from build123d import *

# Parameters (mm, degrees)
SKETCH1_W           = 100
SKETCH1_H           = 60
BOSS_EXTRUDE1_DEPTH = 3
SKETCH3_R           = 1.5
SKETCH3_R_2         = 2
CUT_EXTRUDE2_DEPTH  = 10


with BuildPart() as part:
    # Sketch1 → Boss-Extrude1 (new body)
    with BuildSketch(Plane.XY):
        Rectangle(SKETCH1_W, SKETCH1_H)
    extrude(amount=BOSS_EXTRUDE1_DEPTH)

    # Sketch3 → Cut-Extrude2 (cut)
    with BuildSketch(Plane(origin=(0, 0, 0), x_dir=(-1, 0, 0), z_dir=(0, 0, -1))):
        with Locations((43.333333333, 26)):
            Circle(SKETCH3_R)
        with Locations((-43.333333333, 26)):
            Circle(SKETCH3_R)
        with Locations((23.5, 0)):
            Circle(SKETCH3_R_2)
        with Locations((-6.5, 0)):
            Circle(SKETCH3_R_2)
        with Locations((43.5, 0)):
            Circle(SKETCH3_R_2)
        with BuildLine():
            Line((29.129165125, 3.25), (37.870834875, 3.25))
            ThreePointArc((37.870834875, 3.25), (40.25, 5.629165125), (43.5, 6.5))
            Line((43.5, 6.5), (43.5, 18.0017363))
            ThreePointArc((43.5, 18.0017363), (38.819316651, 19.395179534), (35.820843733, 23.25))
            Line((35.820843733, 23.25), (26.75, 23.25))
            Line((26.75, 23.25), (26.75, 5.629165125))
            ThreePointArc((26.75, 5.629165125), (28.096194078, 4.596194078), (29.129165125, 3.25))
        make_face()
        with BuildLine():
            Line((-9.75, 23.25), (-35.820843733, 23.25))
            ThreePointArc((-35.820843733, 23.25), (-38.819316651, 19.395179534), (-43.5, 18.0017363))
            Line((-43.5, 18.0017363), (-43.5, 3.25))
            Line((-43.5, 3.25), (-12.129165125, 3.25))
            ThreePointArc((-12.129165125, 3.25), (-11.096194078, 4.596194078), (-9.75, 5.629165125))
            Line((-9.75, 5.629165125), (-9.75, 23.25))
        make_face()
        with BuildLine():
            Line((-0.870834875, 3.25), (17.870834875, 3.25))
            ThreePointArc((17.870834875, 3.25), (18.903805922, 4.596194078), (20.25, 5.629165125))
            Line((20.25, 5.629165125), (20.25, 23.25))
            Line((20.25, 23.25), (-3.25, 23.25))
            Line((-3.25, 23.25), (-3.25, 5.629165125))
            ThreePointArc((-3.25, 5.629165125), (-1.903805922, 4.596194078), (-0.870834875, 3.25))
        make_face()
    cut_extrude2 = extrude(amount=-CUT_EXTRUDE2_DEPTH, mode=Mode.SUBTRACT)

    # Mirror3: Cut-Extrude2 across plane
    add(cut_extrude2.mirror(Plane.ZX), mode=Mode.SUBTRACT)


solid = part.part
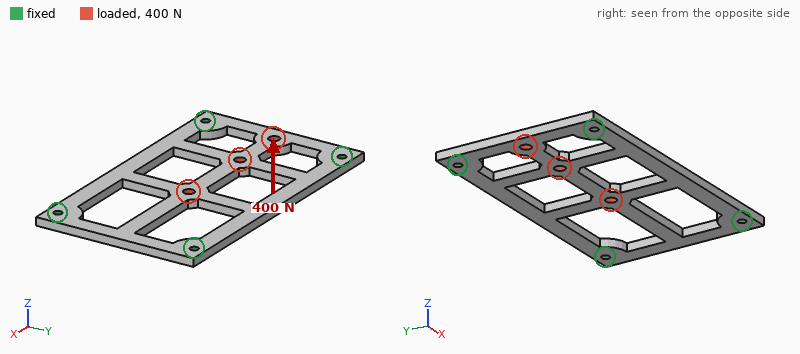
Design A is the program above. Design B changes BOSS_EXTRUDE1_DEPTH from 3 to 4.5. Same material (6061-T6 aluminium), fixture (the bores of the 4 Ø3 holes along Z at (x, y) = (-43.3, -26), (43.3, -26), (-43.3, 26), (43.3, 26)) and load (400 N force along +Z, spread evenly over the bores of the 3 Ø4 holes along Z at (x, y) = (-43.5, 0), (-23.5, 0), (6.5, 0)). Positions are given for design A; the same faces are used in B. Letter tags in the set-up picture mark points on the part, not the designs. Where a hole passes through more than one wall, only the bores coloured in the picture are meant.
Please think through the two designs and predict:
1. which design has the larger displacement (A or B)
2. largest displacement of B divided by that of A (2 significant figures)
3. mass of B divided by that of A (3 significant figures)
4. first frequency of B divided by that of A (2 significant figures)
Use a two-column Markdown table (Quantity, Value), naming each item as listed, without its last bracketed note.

| Quantity | Value |
|---|---|
| which design has the larger displacement | A |
| largest displacement of B divided by that of A | 0.32 |
| mass of B divided by that of A | 1.50 |
| first frequency of B divided by that of A | 1.4 |
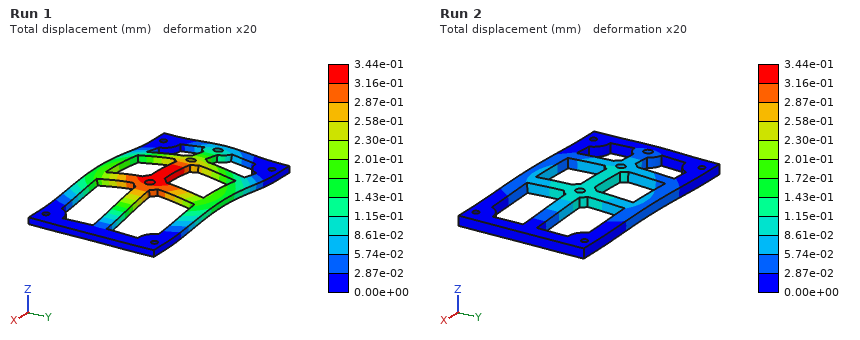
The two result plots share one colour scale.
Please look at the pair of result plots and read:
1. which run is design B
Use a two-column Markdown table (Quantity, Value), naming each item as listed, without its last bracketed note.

| Quantity | Value |
|---|---|
| which run is design B | Run 2 |
